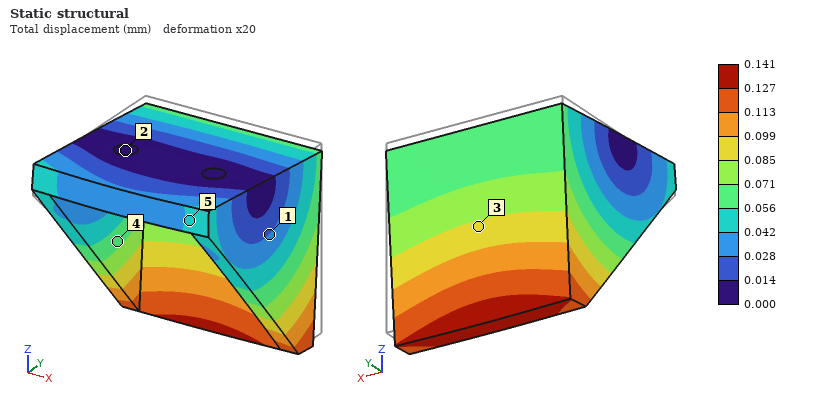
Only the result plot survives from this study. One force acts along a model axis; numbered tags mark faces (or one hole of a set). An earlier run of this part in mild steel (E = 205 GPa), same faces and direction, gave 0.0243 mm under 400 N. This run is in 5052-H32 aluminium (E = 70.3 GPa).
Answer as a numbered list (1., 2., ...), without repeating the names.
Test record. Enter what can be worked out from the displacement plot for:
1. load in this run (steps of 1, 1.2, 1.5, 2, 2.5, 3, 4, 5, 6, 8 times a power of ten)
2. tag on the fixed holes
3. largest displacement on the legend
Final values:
1. 800 N
2. 2
3. 0.141 mm
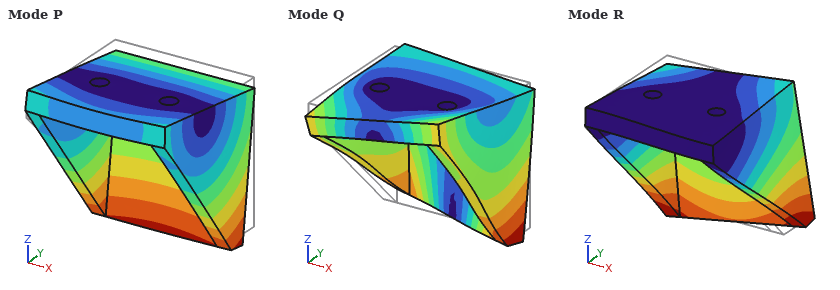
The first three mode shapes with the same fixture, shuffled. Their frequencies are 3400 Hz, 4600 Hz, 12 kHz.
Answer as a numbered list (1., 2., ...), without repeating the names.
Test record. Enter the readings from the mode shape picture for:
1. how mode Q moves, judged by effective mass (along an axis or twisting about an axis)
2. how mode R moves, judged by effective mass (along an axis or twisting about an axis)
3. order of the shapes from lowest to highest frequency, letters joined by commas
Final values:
1. along X
2. along X
3. P, R, Q
